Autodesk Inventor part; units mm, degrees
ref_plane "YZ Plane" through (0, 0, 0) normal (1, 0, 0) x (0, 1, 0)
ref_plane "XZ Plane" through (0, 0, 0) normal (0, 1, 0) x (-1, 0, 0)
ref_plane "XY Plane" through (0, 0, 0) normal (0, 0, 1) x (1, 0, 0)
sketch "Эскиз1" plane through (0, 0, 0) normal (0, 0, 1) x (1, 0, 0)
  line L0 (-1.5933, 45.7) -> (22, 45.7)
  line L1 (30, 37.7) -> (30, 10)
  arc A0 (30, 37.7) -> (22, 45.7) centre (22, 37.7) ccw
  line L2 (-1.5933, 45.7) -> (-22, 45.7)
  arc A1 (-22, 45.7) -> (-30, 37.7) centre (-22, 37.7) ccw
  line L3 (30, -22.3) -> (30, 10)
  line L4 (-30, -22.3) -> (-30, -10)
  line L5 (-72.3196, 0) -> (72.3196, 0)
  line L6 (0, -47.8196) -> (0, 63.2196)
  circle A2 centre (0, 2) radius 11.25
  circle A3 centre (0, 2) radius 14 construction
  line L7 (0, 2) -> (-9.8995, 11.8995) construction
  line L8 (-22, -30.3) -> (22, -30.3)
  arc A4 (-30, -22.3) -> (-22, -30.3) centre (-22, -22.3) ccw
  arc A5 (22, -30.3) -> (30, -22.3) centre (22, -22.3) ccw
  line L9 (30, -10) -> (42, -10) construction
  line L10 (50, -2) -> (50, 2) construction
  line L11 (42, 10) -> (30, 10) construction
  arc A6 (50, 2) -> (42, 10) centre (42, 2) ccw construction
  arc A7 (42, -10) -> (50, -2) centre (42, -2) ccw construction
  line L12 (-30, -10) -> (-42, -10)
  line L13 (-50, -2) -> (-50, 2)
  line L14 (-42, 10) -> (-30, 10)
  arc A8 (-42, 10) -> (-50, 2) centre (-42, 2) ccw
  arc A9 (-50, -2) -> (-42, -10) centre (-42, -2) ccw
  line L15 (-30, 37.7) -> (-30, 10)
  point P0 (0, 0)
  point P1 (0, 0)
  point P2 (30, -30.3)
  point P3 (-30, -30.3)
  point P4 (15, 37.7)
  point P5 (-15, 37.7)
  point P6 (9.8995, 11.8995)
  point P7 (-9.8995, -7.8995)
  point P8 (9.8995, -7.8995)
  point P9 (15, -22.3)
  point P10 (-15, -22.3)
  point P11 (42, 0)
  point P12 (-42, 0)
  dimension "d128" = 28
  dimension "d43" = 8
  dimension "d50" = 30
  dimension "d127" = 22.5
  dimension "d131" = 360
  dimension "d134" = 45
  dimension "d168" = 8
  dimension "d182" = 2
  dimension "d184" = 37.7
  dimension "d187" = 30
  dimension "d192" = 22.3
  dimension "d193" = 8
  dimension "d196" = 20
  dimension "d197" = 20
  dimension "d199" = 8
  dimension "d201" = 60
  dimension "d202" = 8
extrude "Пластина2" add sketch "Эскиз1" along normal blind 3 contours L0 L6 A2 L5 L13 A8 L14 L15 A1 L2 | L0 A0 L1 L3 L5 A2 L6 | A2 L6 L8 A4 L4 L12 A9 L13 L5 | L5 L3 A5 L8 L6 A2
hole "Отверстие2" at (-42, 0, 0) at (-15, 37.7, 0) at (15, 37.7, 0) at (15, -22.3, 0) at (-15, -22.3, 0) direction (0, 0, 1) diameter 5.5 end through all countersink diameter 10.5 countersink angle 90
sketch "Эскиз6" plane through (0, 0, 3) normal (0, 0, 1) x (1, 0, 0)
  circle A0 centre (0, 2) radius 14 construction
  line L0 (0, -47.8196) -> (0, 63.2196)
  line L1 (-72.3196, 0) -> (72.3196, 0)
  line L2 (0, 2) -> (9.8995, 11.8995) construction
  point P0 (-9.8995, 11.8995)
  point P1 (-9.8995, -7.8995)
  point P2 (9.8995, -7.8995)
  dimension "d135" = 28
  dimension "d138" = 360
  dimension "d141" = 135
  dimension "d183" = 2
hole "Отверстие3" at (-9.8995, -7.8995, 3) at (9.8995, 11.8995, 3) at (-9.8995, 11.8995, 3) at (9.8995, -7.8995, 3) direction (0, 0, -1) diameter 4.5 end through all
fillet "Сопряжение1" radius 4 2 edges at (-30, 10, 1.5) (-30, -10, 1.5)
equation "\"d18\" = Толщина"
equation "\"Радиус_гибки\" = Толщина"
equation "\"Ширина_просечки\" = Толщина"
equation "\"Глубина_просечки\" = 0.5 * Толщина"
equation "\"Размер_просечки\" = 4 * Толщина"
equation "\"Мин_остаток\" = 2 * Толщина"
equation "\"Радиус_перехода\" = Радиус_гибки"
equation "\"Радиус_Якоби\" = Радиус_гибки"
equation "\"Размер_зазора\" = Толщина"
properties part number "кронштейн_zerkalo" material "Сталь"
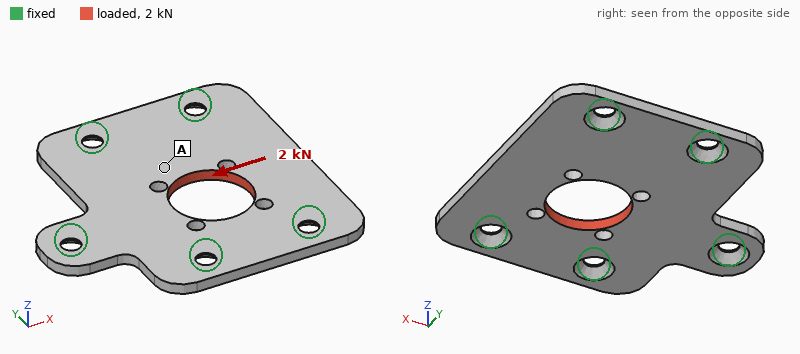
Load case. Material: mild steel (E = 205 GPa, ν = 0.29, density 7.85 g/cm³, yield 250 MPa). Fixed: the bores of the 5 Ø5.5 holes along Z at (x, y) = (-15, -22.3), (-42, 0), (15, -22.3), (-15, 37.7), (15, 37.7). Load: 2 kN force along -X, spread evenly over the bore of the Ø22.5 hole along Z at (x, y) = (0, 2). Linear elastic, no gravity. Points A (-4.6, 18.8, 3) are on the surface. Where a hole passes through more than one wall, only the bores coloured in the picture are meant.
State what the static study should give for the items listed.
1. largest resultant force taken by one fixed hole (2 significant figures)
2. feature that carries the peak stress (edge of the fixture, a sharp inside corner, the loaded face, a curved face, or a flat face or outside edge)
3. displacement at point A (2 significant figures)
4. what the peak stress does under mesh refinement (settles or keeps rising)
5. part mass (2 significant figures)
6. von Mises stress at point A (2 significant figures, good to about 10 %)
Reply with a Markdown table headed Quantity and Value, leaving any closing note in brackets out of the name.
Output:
| Quantity | Value |
|---|---|
| largest resultant force taken by one fixed hole | 450 N |
| feature that carries the peak stress | edge of the fixture |
| displacement at point A | 2.4 µm |
| what the peak stress does under mesh refinement | keeps rising |
| part mass | 99 g |
| von Mises stress at point A | 9.5 MPa |
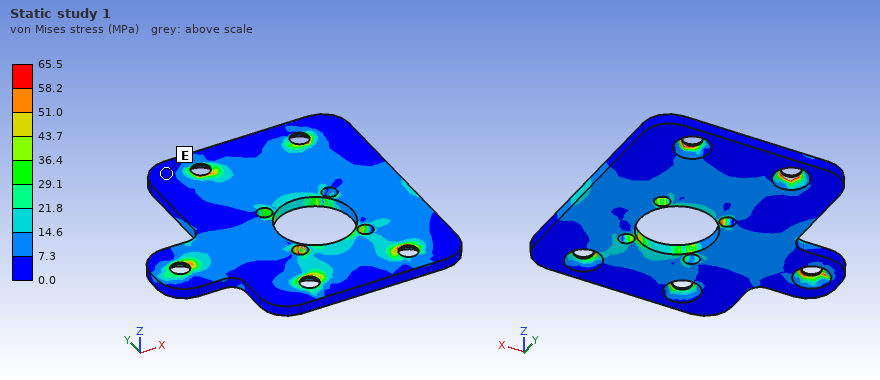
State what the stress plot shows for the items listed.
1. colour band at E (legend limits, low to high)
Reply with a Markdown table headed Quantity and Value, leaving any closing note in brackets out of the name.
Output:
| Quantity | Value |
|---|---|
| colour band at E | 0.0 to 7.3 MPa |
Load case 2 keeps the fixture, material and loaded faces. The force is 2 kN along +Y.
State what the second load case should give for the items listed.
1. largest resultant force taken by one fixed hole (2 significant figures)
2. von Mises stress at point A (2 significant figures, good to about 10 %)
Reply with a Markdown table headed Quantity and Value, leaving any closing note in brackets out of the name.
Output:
| Quantity | Value |
|---|---|
| largest resultant force taken by one fixed hole | 540 N |
| von Mises stress at point A | 12 MPa |
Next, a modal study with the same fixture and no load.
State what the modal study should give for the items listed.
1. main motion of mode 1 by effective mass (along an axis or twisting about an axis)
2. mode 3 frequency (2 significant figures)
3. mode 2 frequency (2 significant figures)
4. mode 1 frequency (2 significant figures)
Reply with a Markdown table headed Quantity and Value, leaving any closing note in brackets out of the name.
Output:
| Quantity | Value |
|---|---|
| main motion of mode 1 by effective mass | along Z |
| mode 3 frequency | 7500 Hz |
| mode 2 frequency | 4900 Hz |
| mode 1 frequency | 3400 Hz |
